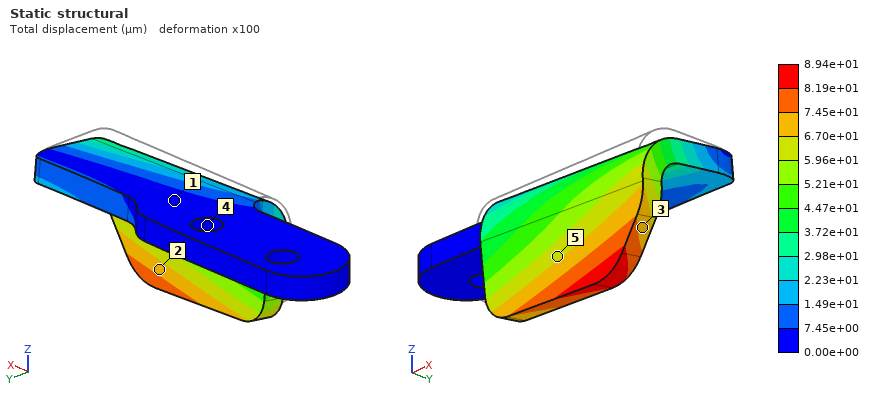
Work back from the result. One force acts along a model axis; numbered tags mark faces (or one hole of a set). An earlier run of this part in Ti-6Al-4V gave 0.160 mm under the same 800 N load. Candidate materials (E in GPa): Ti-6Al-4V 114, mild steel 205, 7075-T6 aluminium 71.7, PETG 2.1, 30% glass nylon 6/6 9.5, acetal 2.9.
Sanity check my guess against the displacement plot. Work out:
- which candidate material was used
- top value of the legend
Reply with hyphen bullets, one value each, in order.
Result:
- mild steel
- 8.94e+01 µm
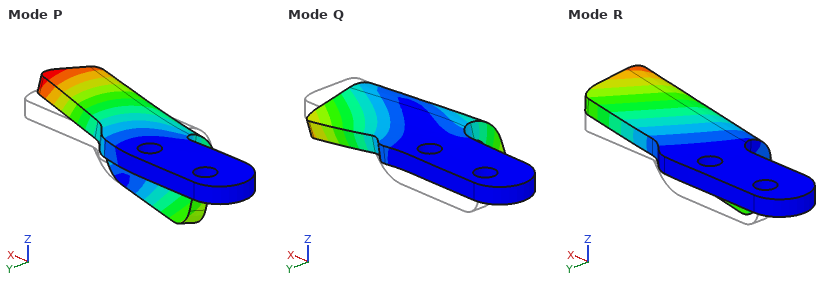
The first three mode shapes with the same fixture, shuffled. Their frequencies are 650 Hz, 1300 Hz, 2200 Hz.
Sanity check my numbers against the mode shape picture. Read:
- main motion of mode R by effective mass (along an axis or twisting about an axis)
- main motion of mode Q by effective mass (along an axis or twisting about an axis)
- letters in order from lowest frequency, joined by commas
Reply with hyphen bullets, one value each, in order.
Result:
- along Z
- along Y
- R, Q, P
